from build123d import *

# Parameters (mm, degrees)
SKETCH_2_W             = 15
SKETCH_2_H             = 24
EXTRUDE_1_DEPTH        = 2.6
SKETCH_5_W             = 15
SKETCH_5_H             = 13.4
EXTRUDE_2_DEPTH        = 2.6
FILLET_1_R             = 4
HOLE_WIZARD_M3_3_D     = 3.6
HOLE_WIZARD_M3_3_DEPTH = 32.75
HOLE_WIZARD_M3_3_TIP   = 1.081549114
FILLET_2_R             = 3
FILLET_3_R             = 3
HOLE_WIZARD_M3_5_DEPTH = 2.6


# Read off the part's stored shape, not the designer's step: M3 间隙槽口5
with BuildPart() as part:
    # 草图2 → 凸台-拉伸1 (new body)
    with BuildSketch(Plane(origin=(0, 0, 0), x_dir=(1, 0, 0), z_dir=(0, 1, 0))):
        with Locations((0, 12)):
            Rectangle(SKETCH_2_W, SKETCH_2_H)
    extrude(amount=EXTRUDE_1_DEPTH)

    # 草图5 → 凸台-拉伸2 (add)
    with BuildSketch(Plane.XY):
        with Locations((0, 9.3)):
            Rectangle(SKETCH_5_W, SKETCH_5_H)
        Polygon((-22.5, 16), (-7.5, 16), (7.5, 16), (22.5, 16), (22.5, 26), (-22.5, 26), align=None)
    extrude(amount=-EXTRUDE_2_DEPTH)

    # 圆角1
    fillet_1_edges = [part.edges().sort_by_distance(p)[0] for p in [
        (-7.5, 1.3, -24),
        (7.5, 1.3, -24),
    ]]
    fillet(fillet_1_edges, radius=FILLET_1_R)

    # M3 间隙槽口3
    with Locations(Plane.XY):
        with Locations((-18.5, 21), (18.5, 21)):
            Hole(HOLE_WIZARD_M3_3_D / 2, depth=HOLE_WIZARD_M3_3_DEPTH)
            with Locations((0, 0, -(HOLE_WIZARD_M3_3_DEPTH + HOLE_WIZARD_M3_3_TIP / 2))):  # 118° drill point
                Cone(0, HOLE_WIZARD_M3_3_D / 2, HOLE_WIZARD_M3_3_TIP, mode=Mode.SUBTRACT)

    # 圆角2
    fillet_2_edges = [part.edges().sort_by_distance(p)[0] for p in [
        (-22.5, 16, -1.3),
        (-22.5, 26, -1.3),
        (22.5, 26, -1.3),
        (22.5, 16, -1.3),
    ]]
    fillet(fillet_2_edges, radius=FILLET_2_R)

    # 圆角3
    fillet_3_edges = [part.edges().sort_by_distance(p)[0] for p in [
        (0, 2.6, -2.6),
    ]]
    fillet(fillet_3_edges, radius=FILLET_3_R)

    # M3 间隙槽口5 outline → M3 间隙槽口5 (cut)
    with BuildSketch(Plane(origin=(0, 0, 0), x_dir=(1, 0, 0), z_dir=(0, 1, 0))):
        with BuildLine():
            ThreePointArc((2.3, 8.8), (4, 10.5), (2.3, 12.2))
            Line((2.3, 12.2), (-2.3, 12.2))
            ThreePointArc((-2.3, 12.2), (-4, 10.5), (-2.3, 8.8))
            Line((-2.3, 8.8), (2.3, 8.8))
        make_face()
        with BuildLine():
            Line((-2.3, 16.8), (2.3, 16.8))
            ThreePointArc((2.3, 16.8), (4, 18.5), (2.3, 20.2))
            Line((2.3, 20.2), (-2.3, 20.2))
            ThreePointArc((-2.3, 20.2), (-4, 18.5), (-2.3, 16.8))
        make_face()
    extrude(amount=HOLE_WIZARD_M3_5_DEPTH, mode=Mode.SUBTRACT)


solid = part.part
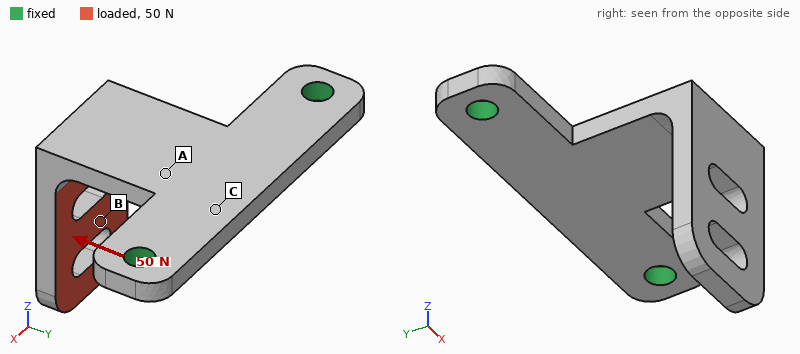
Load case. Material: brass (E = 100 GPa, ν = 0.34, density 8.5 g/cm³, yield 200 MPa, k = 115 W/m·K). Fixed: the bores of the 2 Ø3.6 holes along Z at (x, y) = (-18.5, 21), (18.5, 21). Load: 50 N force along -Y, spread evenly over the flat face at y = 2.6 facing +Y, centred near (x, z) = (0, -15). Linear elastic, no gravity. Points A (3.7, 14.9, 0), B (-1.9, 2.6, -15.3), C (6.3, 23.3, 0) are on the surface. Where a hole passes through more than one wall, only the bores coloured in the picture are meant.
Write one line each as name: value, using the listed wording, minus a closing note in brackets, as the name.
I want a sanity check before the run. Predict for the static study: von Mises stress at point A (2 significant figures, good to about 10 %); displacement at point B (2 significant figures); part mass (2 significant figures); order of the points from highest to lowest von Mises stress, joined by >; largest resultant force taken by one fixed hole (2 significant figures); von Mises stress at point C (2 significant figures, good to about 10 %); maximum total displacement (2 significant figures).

von Mises stress at point A: 37 MPa
displacement at point B: 0.13 mm
part mass: 21 g
order of the points from highest to lowest von Mises stress, joined by >: A > C > B
largest resultant force taken by one fixed hole: 26 N
von Mises stress at point C: 16 MPa
maximum total displacement: 0.21 mm
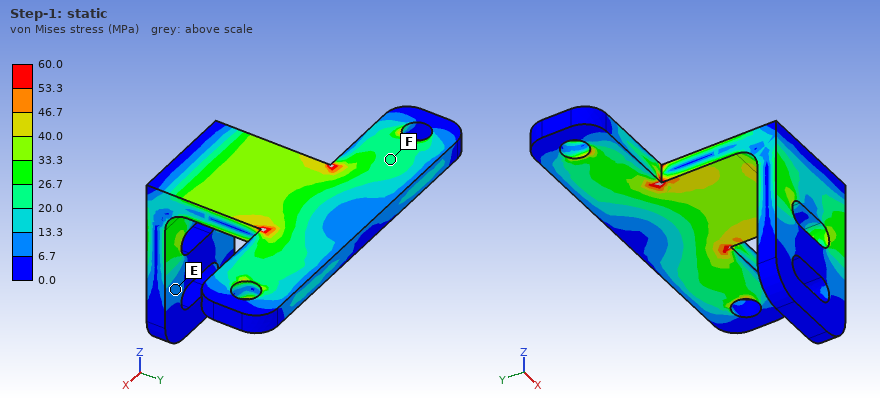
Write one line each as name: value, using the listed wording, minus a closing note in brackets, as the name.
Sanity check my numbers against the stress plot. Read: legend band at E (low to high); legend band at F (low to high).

legend band at E: 6.7 to 13.3 MPa
legend band at F: 20.0 to 26.7 MPa
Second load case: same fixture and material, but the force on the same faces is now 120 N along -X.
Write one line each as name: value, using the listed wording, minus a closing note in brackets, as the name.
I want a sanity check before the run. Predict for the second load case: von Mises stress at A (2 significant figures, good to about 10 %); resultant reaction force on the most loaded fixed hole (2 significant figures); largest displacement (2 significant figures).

von Mises stress at A: 67 MPa
resultant reaction force on the most loaded fixed hole: 110 N
largest displacement: 0.18 mm
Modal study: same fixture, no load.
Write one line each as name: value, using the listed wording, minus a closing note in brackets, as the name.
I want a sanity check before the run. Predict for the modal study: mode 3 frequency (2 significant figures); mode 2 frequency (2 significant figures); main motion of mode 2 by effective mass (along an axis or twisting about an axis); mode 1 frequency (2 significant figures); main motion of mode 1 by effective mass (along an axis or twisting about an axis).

mode 3 frequency: 2700 Hz
mode 2 frequency: 2100 Hz
main motion of mode 2 by effective mass: along X
mode 1 frequency: 970 Hz
main motion of mode 1 by effective mass: along Z
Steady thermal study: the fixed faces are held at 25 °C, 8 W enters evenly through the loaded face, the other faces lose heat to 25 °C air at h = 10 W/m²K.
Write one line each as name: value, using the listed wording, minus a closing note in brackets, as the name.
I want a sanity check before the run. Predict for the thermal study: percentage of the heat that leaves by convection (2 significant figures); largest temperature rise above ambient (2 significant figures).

percentage of the heat that leaves by convection: 7.5 %
largest temperature rise above ambient: 75 K
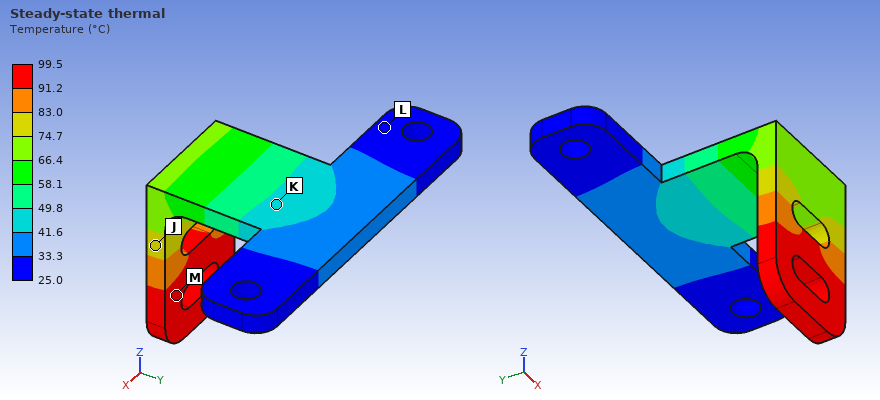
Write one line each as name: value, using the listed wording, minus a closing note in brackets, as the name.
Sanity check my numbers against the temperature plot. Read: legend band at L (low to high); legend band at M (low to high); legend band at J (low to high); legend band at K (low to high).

legend band at L: 25.0 to 33.3 °C
legend band at M: 91.2 to 99.5 °C
legend band at J: 74.7 to 83.0 °C
legend band at K: 41.6 to 49.8 °C
